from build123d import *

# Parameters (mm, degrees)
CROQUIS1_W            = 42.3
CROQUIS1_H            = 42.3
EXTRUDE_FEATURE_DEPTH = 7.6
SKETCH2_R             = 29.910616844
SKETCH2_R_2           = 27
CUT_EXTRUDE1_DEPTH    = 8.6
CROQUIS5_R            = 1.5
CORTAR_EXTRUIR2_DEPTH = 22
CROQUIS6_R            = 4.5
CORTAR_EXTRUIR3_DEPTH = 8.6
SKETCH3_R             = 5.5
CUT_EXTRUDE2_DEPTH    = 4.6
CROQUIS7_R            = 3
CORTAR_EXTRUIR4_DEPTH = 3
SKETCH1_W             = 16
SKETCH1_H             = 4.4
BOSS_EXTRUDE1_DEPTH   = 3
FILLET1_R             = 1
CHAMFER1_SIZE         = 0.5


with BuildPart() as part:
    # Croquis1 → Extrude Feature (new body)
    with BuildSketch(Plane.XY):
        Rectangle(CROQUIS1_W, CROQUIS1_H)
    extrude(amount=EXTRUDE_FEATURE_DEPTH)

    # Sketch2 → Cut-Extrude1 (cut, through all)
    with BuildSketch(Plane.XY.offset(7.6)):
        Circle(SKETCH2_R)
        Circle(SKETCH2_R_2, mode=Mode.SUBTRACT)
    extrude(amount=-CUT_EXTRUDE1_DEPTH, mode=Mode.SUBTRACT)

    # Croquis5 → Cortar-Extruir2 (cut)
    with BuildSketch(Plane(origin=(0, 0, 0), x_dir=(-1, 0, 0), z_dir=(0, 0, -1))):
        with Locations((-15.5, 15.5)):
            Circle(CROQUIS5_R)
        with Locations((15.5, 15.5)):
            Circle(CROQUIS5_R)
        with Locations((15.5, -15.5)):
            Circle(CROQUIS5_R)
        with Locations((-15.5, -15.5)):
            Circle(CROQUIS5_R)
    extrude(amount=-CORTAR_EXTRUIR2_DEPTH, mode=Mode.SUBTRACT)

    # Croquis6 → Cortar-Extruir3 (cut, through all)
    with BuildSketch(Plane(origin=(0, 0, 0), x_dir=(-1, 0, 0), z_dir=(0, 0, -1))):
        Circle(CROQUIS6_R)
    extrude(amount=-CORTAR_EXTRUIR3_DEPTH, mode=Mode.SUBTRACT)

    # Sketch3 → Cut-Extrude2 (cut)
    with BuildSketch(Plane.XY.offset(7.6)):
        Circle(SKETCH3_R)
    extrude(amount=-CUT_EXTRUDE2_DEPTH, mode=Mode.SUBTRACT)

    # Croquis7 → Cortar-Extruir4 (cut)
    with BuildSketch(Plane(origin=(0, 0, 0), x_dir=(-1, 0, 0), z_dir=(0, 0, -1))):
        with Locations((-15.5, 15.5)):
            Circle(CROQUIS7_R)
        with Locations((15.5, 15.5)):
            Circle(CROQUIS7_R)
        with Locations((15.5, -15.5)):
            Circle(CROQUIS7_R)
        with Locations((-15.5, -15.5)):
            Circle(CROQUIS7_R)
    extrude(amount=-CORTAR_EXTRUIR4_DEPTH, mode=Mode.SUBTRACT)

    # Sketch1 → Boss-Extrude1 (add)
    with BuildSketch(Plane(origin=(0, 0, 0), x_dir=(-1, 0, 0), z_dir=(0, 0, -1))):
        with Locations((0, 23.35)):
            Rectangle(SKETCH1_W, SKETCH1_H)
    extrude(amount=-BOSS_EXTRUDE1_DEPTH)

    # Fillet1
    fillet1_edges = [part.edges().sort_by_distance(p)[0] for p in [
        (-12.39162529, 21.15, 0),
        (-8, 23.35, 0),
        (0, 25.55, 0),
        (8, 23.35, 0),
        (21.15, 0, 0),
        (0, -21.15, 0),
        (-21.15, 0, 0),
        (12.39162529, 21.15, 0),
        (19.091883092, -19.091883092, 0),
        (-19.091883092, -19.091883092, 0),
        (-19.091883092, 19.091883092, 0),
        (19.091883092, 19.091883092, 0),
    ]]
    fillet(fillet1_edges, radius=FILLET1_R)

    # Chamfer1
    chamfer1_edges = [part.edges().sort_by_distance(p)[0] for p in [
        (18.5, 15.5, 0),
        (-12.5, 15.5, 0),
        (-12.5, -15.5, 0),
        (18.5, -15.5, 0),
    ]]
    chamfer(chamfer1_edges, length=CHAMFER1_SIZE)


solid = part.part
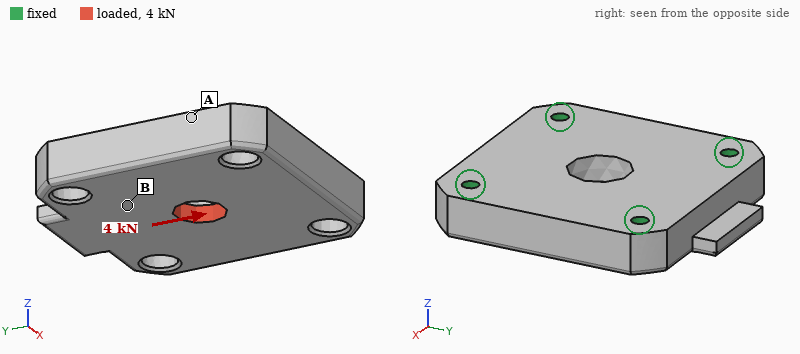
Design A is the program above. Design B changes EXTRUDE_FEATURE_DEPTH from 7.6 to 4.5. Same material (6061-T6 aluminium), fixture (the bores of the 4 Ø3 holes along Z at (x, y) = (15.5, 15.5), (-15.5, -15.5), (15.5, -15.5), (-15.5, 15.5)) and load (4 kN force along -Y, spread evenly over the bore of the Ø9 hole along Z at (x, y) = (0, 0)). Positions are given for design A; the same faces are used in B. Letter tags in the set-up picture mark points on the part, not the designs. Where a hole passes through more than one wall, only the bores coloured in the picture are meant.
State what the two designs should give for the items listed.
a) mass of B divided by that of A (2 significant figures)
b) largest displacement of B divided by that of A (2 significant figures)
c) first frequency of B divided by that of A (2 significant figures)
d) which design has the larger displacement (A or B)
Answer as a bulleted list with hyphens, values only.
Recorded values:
- 0.59
- 1.5
- 0.63
- B
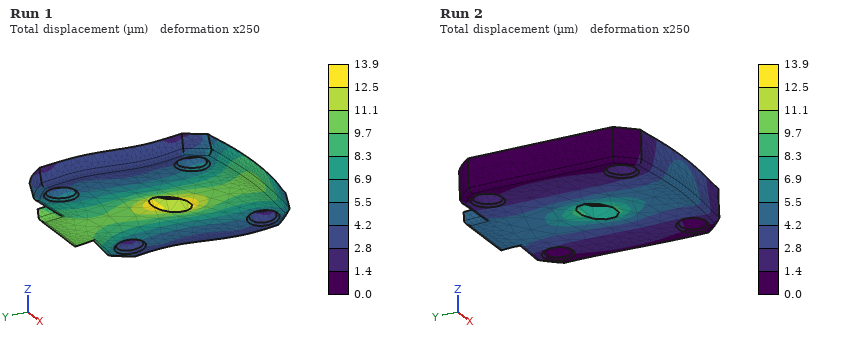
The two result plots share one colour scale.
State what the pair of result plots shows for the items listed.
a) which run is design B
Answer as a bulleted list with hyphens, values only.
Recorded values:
- Run 1
